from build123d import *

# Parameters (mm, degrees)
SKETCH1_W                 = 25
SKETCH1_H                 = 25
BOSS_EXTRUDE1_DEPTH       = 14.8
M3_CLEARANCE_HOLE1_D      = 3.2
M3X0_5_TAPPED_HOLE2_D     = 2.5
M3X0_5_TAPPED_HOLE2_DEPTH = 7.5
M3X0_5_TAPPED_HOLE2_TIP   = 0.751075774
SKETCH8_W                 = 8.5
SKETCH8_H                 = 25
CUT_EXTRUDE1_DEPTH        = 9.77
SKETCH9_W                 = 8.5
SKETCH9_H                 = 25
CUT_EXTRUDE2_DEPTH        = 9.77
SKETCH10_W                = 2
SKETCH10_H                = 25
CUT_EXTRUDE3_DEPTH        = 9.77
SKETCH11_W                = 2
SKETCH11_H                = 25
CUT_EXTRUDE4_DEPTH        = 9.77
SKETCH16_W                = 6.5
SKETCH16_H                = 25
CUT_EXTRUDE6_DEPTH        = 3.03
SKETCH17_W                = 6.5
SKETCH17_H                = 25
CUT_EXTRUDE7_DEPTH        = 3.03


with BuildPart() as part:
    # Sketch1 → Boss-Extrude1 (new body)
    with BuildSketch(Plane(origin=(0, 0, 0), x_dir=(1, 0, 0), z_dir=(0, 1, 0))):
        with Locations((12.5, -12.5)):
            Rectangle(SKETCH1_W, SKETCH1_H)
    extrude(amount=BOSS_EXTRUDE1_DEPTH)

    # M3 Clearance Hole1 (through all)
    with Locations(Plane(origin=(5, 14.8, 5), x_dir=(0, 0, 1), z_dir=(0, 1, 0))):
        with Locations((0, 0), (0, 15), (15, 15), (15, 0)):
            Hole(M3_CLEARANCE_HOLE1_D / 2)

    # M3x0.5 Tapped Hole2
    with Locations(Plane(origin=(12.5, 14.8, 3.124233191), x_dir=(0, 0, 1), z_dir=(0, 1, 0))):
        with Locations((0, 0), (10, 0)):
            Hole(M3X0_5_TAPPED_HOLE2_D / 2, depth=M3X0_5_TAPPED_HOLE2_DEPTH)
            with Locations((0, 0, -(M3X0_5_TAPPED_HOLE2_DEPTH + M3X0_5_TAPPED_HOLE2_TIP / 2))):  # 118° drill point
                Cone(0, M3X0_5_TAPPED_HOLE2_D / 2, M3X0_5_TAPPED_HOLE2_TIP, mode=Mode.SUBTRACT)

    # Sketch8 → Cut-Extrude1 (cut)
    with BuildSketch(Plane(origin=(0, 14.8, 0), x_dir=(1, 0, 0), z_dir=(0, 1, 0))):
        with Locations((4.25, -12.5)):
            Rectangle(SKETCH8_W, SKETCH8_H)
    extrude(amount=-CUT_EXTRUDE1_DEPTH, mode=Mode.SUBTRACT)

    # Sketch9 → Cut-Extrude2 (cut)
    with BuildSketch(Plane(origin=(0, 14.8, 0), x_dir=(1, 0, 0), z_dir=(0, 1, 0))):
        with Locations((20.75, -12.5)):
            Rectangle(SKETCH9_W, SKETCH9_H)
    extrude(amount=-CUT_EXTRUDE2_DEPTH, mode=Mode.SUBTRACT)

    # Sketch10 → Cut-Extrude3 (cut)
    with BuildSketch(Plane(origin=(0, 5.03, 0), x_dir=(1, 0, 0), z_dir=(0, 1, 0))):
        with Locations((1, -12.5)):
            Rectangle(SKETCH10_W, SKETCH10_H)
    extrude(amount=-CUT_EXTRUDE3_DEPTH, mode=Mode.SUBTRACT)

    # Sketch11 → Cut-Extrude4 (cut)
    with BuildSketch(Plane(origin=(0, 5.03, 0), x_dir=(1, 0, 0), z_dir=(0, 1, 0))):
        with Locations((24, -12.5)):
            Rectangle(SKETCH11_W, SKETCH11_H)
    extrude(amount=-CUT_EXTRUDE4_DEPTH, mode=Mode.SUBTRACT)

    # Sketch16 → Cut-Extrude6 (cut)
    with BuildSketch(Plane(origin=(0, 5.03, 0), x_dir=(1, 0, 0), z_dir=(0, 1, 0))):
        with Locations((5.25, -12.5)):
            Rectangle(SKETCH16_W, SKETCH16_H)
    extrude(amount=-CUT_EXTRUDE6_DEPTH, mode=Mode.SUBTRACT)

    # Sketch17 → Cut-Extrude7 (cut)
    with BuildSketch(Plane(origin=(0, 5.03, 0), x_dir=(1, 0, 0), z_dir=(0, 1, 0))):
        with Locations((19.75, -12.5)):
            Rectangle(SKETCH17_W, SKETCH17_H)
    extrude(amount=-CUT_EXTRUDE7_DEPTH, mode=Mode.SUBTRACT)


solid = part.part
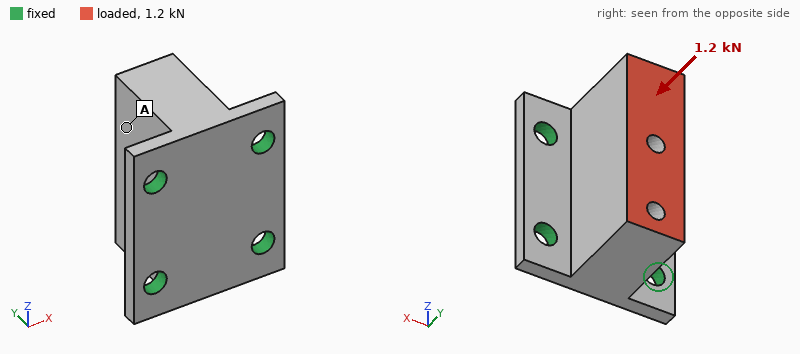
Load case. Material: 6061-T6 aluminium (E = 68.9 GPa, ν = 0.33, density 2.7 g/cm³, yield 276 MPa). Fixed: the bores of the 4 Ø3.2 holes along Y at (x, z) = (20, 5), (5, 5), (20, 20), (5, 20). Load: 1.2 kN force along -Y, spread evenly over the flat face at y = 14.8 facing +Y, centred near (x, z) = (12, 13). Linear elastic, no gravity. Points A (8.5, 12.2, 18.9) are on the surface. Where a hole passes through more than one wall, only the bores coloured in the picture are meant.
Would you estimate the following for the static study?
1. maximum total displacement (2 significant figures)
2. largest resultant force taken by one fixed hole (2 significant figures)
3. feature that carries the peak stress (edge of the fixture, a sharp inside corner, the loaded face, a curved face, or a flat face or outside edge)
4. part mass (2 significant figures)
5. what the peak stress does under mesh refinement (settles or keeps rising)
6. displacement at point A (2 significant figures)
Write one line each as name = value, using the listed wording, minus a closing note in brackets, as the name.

maximum total displacement = 6.8 µm
largest resultant force taken by one fixed hole = 330 N
feature that carries the peak stress = edge of the fixture
part mass = 9.4 g
what the peak stress does under mesh refinement = keeps rising
displacement at point A = 6.5 µm
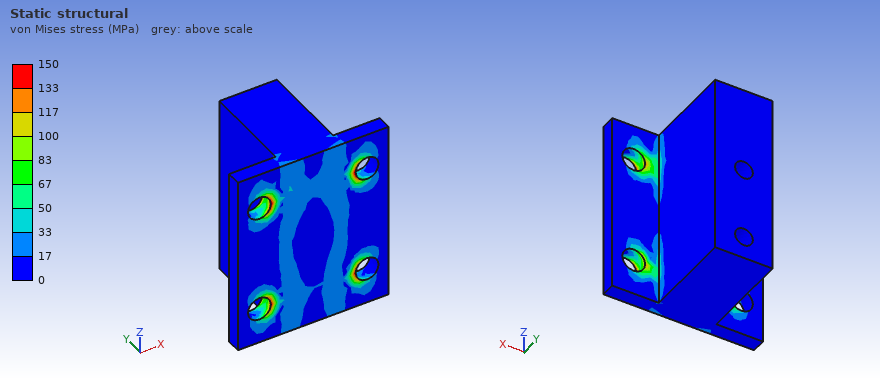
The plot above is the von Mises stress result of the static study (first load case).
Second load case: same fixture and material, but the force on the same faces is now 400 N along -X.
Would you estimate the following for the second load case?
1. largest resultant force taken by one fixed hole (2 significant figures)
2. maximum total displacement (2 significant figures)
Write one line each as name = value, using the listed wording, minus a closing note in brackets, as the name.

largest resultant force taken by one fixed hole = 270 N
maximum total displacement = 17 µm
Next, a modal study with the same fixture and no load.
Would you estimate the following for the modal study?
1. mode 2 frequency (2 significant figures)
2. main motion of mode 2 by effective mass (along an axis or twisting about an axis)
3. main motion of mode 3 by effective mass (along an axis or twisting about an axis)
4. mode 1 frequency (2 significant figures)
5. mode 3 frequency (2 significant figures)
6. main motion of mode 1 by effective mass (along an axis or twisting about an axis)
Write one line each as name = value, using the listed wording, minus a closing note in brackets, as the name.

mode 2 frequency = 18 kHz
main motion of mode 2 by effective mass = along Z
main motion of mode 3 by effective mass = along Y
mode 1 frequency = 16 kHz
mode 3 frequency = 26 kHz
main motion of mode 1 by effective mass = along X
